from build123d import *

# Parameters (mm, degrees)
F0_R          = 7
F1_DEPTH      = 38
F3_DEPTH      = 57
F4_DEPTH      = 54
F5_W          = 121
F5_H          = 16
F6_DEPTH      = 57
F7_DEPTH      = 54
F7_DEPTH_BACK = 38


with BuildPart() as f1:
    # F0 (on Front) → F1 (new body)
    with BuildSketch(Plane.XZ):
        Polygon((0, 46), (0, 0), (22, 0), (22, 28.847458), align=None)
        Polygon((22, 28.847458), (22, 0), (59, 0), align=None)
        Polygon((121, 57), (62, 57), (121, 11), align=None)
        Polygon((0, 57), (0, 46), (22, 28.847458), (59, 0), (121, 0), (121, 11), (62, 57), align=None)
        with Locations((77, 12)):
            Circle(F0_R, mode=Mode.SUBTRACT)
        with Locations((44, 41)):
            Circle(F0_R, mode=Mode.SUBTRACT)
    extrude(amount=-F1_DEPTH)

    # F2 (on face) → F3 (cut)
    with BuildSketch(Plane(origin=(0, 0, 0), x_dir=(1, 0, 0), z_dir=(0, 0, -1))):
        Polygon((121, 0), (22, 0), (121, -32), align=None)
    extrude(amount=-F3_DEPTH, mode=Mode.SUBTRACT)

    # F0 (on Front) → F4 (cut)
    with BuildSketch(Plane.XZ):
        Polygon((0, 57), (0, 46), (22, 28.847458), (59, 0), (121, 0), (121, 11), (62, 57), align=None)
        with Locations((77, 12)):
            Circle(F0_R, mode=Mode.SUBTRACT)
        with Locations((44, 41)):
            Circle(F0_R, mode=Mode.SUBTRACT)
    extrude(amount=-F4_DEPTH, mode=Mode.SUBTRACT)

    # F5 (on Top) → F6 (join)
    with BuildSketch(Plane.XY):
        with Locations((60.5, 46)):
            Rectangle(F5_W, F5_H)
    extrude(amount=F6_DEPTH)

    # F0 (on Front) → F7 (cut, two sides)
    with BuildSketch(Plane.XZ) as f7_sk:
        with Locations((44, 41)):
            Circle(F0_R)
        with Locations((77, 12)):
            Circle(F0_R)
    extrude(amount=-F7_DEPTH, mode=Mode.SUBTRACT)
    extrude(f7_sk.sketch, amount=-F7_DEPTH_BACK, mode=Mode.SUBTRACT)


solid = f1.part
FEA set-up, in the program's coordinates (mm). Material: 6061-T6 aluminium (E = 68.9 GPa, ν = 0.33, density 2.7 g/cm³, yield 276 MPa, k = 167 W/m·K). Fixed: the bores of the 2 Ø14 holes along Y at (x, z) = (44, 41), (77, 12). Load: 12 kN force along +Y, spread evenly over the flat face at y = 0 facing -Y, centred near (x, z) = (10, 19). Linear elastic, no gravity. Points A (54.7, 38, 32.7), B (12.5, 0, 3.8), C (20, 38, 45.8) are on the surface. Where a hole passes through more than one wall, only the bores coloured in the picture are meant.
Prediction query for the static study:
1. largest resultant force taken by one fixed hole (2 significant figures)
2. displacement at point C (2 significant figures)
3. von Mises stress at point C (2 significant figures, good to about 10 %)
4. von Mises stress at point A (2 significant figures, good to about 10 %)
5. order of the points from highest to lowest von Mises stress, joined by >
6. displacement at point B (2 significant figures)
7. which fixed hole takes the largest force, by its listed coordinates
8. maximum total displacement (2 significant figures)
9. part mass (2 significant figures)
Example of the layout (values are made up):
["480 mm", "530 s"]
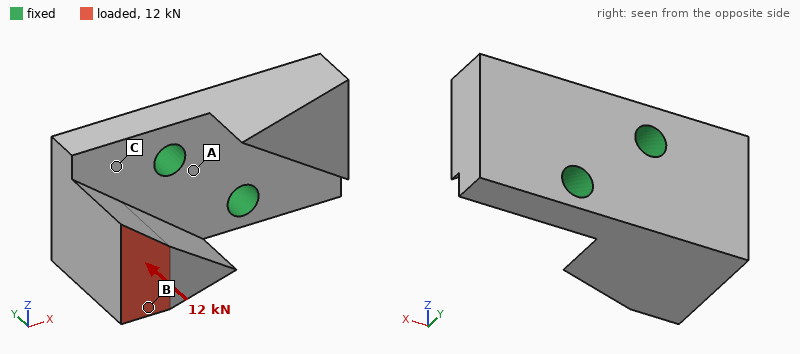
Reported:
["13 kN", "0.061 mm", "71 MPa", "44 MPa", "C > A > B", "0.35 mm", "(44, 41)", "0.40 mm", "460 g"]
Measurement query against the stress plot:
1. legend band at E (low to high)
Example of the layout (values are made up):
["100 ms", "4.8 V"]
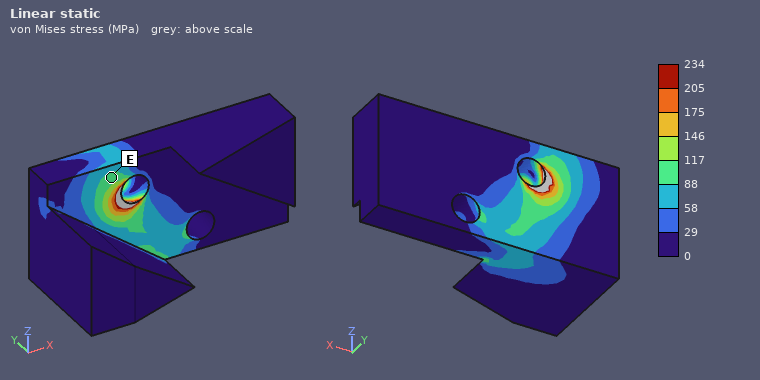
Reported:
["88 to 117 MPa"]
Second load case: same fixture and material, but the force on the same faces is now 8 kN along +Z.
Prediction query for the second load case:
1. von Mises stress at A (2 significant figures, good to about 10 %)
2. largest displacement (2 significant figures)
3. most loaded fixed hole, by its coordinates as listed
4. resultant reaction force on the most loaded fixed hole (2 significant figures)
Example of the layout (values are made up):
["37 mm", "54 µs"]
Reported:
["39 MPa", "0.39 mm", "(44, 41)", "11 kN"]
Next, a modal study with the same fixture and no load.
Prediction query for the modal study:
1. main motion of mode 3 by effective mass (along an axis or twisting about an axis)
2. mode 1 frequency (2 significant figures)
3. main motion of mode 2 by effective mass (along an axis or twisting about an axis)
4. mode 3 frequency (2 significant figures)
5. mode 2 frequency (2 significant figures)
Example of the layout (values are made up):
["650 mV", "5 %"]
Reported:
["along Z", "2400 Hz", "along Y", "4600 Hz", "4000 Hz"]
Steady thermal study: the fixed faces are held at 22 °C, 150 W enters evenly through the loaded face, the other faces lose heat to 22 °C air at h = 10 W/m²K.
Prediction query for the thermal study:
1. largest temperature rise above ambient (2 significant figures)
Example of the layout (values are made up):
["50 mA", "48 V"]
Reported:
["62 K"]
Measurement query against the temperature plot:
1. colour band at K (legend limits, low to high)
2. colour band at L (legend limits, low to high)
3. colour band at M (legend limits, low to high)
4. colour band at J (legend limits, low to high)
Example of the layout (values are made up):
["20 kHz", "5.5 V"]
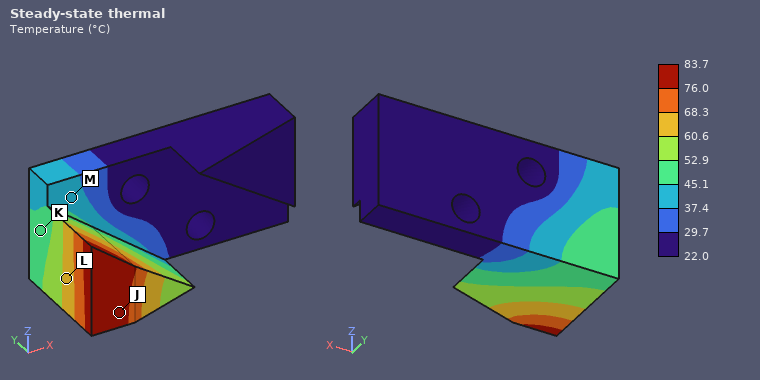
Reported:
["45.1 to 52.9 °C", "60.6 to 68.3 °C", "37.4 to 45.1 °C", "76.0 to 83.7 °C"]
